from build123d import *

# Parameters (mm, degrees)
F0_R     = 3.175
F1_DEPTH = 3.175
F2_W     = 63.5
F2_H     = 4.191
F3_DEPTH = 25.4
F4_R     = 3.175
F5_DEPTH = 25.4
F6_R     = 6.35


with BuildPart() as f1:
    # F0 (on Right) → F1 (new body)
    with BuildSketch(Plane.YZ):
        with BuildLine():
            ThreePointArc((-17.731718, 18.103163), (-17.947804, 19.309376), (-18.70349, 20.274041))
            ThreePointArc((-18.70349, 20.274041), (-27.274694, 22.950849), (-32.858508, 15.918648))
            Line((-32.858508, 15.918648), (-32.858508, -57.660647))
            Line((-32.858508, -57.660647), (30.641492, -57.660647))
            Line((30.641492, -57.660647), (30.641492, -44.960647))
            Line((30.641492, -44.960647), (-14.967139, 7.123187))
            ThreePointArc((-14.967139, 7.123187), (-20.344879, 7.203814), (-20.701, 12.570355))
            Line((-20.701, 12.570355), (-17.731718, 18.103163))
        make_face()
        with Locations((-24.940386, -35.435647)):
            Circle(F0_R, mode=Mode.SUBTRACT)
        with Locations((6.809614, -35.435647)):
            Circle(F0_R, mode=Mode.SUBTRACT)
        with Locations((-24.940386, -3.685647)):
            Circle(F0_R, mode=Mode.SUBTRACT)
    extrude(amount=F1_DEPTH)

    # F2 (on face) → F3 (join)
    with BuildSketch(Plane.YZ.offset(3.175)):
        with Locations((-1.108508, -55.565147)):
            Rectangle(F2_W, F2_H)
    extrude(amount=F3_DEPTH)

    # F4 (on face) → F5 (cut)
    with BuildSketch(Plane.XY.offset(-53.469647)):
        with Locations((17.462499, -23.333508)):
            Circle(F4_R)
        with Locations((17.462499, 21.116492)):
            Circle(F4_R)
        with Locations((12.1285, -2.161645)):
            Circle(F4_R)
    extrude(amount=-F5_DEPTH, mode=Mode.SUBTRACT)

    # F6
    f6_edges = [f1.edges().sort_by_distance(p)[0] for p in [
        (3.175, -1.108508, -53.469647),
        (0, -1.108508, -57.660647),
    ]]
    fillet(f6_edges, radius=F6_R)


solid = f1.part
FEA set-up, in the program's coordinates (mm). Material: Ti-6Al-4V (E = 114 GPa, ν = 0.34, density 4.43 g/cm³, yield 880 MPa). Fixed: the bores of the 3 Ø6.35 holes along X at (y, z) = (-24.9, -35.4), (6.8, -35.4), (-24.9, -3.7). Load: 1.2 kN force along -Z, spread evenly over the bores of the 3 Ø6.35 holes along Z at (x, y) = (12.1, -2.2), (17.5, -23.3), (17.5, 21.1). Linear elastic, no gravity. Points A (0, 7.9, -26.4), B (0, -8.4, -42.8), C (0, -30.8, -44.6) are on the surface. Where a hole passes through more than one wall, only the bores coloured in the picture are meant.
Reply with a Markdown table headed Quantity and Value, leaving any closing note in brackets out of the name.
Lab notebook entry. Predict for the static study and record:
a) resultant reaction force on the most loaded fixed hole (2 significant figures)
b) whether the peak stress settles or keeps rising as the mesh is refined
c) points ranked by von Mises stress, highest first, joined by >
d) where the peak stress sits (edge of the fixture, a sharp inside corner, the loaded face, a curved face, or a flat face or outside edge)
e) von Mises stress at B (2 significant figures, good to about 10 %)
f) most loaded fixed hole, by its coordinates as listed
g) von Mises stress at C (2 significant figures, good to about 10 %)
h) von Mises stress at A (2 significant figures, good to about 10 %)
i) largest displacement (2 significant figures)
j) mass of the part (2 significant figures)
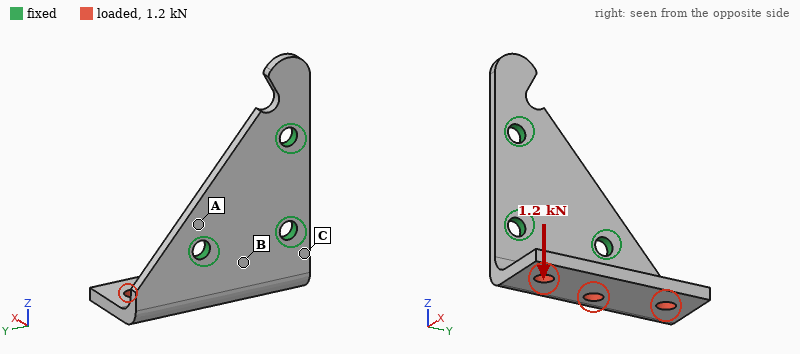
| Quantity | Value |
|---|---|
| resultant reaction force on the most loaded fixed hole | 800 N |
| whether the peak stress settles or keeps rising as the mesh is refined | keeps rising |
| points ranked by von Mises stress, highest first, joined by > | C > B > A |
| where the peak stress sits | edge of the fixture |
| von Mises stress at B | 130 MPa |
| most loaded fixed hole, by its coordinates as listed | (6.8, -35.4) |
| von Mises stress at C | 170 MPa |
| von Mises stress at A | 39 MPa |
| largest displacement | 0.46 mm |
| mass of the part | 71 g |
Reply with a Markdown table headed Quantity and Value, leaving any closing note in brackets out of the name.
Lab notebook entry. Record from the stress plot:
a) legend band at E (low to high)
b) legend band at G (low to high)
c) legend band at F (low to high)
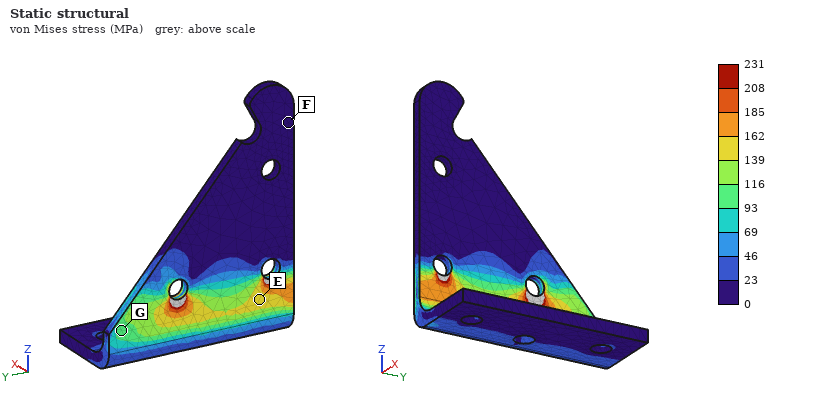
| Quantity | Value |
|---|---|
| legend band at E | 139 to 162 MPa |
| legend band at G | 93 to 116 MPa |
| legend band at F | 0 to 23 MPa |
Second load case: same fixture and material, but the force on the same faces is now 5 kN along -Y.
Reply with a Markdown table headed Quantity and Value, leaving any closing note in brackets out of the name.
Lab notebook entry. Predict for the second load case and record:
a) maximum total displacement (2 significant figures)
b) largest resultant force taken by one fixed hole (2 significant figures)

| Quantity | Value |
|---|---|
| maximum total displacement | 0.52 mm |
| largest resultant force taken by one fixed hole | 4.2 kN |
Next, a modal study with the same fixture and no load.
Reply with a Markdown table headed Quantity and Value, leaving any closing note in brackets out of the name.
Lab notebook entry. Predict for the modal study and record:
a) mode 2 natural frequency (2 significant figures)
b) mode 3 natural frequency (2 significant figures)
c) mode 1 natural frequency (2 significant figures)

| Quantity | Value |
|---|---|
| mode 2 natural frequency | 2800 Hz |
| mode 3 natural frequency | 4800 Hz |
| mode 1 natural frequency | 1600 Hz |
